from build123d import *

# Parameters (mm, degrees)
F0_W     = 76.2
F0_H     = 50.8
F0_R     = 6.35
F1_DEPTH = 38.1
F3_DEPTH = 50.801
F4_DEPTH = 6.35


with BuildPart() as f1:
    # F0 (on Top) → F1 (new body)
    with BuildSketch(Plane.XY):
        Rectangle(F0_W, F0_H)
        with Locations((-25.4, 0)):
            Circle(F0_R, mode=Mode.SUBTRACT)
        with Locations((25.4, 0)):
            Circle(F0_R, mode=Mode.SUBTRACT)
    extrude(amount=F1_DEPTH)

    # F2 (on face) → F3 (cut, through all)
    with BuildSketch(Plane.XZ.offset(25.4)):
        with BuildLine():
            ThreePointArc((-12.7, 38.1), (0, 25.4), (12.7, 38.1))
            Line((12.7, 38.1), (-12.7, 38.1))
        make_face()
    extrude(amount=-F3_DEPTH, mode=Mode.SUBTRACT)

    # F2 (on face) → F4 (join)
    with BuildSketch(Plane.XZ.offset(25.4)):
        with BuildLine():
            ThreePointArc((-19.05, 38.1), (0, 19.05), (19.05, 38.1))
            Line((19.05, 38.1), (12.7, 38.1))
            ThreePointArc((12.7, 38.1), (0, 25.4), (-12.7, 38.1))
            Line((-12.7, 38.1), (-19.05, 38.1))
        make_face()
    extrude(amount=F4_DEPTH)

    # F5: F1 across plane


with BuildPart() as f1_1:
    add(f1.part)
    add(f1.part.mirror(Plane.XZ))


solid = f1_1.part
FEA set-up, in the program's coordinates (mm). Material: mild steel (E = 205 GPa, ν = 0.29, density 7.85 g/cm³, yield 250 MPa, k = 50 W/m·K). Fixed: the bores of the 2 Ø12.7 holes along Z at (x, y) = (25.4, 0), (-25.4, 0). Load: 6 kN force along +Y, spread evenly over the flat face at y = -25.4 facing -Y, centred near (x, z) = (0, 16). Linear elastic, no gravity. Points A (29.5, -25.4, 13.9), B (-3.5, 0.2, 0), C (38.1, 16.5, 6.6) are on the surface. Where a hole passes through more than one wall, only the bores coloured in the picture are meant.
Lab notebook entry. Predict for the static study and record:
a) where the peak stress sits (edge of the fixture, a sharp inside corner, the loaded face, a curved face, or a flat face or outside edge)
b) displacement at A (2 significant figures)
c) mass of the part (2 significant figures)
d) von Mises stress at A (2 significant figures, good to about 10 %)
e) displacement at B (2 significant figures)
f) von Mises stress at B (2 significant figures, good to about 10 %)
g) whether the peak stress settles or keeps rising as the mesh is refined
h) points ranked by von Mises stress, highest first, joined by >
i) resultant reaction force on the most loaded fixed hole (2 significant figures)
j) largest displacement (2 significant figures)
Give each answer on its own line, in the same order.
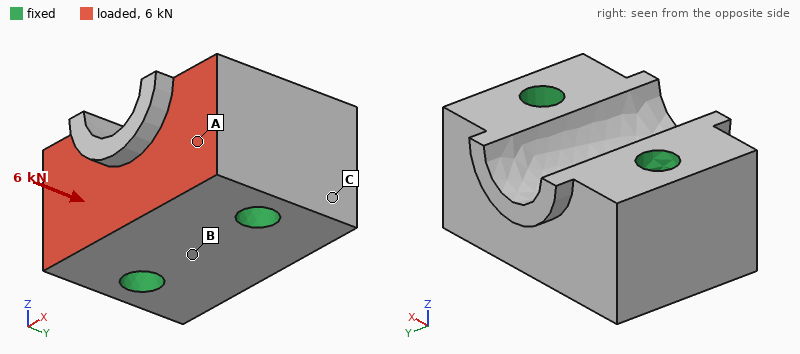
edge of the fixture
0.30 µm
1.0 kg
2.8 MPa
0.22 µm
1.2 MPa
keeps rising
A > B > C
3.0 kN
0.49 µm
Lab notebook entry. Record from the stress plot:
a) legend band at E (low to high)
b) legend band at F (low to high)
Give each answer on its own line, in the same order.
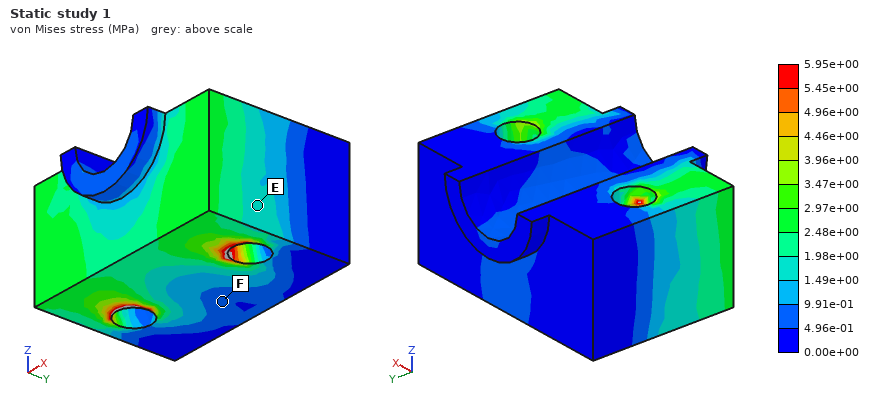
1.49e+00 to 1.98e+00 MPa
4.96e-01 to 9.91e-01 MPa
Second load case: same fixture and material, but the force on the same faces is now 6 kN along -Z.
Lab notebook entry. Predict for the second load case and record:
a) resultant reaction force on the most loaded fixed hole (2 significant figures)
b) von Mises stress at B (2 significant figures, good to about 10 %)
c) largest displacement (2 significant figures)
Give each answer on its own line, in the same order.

3.0 kN
3.2 MPa
1.8 µm
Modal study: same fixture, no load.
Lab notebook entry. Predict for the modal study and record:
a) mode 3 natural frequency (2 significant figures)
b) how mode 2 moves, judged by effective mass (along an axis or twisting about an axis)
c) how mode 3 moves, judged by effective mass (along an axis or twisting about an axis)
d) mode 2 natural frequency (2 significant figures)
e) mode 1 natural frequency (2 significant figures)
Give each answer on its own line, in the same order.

26 kHz
along Z
twisting about Z
24 kHz
22 kHz
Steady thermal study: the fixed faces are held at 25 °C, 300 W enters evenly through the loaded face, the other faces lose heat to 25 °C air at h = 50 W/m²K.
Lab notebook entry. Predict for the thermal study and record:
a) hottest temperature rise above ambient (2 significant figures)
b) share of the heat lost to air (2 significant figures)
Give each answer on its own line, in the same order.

59 K
3.6 %
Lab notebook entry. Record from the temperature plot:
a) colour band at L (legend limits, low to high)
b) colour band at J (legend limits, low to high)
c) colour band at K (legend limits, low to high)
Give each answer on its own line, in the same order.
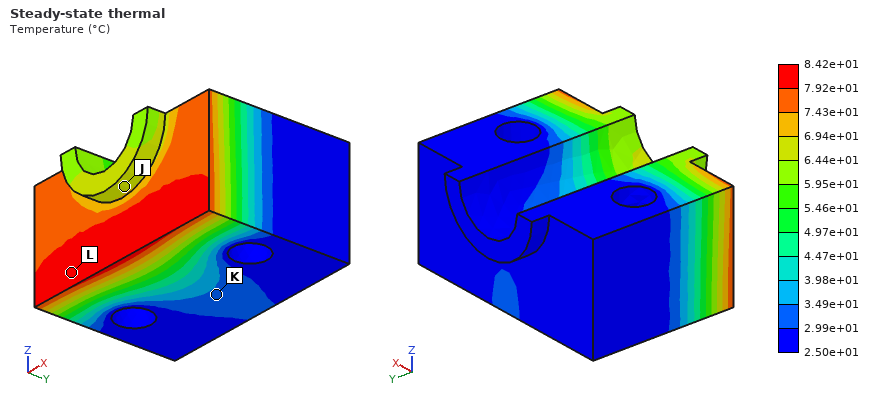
7.92e+01 to 8.42e+01 °C
6.44e+01 to 6.94e+01 °C
2.99e+01 to 3.49e+01 °C
